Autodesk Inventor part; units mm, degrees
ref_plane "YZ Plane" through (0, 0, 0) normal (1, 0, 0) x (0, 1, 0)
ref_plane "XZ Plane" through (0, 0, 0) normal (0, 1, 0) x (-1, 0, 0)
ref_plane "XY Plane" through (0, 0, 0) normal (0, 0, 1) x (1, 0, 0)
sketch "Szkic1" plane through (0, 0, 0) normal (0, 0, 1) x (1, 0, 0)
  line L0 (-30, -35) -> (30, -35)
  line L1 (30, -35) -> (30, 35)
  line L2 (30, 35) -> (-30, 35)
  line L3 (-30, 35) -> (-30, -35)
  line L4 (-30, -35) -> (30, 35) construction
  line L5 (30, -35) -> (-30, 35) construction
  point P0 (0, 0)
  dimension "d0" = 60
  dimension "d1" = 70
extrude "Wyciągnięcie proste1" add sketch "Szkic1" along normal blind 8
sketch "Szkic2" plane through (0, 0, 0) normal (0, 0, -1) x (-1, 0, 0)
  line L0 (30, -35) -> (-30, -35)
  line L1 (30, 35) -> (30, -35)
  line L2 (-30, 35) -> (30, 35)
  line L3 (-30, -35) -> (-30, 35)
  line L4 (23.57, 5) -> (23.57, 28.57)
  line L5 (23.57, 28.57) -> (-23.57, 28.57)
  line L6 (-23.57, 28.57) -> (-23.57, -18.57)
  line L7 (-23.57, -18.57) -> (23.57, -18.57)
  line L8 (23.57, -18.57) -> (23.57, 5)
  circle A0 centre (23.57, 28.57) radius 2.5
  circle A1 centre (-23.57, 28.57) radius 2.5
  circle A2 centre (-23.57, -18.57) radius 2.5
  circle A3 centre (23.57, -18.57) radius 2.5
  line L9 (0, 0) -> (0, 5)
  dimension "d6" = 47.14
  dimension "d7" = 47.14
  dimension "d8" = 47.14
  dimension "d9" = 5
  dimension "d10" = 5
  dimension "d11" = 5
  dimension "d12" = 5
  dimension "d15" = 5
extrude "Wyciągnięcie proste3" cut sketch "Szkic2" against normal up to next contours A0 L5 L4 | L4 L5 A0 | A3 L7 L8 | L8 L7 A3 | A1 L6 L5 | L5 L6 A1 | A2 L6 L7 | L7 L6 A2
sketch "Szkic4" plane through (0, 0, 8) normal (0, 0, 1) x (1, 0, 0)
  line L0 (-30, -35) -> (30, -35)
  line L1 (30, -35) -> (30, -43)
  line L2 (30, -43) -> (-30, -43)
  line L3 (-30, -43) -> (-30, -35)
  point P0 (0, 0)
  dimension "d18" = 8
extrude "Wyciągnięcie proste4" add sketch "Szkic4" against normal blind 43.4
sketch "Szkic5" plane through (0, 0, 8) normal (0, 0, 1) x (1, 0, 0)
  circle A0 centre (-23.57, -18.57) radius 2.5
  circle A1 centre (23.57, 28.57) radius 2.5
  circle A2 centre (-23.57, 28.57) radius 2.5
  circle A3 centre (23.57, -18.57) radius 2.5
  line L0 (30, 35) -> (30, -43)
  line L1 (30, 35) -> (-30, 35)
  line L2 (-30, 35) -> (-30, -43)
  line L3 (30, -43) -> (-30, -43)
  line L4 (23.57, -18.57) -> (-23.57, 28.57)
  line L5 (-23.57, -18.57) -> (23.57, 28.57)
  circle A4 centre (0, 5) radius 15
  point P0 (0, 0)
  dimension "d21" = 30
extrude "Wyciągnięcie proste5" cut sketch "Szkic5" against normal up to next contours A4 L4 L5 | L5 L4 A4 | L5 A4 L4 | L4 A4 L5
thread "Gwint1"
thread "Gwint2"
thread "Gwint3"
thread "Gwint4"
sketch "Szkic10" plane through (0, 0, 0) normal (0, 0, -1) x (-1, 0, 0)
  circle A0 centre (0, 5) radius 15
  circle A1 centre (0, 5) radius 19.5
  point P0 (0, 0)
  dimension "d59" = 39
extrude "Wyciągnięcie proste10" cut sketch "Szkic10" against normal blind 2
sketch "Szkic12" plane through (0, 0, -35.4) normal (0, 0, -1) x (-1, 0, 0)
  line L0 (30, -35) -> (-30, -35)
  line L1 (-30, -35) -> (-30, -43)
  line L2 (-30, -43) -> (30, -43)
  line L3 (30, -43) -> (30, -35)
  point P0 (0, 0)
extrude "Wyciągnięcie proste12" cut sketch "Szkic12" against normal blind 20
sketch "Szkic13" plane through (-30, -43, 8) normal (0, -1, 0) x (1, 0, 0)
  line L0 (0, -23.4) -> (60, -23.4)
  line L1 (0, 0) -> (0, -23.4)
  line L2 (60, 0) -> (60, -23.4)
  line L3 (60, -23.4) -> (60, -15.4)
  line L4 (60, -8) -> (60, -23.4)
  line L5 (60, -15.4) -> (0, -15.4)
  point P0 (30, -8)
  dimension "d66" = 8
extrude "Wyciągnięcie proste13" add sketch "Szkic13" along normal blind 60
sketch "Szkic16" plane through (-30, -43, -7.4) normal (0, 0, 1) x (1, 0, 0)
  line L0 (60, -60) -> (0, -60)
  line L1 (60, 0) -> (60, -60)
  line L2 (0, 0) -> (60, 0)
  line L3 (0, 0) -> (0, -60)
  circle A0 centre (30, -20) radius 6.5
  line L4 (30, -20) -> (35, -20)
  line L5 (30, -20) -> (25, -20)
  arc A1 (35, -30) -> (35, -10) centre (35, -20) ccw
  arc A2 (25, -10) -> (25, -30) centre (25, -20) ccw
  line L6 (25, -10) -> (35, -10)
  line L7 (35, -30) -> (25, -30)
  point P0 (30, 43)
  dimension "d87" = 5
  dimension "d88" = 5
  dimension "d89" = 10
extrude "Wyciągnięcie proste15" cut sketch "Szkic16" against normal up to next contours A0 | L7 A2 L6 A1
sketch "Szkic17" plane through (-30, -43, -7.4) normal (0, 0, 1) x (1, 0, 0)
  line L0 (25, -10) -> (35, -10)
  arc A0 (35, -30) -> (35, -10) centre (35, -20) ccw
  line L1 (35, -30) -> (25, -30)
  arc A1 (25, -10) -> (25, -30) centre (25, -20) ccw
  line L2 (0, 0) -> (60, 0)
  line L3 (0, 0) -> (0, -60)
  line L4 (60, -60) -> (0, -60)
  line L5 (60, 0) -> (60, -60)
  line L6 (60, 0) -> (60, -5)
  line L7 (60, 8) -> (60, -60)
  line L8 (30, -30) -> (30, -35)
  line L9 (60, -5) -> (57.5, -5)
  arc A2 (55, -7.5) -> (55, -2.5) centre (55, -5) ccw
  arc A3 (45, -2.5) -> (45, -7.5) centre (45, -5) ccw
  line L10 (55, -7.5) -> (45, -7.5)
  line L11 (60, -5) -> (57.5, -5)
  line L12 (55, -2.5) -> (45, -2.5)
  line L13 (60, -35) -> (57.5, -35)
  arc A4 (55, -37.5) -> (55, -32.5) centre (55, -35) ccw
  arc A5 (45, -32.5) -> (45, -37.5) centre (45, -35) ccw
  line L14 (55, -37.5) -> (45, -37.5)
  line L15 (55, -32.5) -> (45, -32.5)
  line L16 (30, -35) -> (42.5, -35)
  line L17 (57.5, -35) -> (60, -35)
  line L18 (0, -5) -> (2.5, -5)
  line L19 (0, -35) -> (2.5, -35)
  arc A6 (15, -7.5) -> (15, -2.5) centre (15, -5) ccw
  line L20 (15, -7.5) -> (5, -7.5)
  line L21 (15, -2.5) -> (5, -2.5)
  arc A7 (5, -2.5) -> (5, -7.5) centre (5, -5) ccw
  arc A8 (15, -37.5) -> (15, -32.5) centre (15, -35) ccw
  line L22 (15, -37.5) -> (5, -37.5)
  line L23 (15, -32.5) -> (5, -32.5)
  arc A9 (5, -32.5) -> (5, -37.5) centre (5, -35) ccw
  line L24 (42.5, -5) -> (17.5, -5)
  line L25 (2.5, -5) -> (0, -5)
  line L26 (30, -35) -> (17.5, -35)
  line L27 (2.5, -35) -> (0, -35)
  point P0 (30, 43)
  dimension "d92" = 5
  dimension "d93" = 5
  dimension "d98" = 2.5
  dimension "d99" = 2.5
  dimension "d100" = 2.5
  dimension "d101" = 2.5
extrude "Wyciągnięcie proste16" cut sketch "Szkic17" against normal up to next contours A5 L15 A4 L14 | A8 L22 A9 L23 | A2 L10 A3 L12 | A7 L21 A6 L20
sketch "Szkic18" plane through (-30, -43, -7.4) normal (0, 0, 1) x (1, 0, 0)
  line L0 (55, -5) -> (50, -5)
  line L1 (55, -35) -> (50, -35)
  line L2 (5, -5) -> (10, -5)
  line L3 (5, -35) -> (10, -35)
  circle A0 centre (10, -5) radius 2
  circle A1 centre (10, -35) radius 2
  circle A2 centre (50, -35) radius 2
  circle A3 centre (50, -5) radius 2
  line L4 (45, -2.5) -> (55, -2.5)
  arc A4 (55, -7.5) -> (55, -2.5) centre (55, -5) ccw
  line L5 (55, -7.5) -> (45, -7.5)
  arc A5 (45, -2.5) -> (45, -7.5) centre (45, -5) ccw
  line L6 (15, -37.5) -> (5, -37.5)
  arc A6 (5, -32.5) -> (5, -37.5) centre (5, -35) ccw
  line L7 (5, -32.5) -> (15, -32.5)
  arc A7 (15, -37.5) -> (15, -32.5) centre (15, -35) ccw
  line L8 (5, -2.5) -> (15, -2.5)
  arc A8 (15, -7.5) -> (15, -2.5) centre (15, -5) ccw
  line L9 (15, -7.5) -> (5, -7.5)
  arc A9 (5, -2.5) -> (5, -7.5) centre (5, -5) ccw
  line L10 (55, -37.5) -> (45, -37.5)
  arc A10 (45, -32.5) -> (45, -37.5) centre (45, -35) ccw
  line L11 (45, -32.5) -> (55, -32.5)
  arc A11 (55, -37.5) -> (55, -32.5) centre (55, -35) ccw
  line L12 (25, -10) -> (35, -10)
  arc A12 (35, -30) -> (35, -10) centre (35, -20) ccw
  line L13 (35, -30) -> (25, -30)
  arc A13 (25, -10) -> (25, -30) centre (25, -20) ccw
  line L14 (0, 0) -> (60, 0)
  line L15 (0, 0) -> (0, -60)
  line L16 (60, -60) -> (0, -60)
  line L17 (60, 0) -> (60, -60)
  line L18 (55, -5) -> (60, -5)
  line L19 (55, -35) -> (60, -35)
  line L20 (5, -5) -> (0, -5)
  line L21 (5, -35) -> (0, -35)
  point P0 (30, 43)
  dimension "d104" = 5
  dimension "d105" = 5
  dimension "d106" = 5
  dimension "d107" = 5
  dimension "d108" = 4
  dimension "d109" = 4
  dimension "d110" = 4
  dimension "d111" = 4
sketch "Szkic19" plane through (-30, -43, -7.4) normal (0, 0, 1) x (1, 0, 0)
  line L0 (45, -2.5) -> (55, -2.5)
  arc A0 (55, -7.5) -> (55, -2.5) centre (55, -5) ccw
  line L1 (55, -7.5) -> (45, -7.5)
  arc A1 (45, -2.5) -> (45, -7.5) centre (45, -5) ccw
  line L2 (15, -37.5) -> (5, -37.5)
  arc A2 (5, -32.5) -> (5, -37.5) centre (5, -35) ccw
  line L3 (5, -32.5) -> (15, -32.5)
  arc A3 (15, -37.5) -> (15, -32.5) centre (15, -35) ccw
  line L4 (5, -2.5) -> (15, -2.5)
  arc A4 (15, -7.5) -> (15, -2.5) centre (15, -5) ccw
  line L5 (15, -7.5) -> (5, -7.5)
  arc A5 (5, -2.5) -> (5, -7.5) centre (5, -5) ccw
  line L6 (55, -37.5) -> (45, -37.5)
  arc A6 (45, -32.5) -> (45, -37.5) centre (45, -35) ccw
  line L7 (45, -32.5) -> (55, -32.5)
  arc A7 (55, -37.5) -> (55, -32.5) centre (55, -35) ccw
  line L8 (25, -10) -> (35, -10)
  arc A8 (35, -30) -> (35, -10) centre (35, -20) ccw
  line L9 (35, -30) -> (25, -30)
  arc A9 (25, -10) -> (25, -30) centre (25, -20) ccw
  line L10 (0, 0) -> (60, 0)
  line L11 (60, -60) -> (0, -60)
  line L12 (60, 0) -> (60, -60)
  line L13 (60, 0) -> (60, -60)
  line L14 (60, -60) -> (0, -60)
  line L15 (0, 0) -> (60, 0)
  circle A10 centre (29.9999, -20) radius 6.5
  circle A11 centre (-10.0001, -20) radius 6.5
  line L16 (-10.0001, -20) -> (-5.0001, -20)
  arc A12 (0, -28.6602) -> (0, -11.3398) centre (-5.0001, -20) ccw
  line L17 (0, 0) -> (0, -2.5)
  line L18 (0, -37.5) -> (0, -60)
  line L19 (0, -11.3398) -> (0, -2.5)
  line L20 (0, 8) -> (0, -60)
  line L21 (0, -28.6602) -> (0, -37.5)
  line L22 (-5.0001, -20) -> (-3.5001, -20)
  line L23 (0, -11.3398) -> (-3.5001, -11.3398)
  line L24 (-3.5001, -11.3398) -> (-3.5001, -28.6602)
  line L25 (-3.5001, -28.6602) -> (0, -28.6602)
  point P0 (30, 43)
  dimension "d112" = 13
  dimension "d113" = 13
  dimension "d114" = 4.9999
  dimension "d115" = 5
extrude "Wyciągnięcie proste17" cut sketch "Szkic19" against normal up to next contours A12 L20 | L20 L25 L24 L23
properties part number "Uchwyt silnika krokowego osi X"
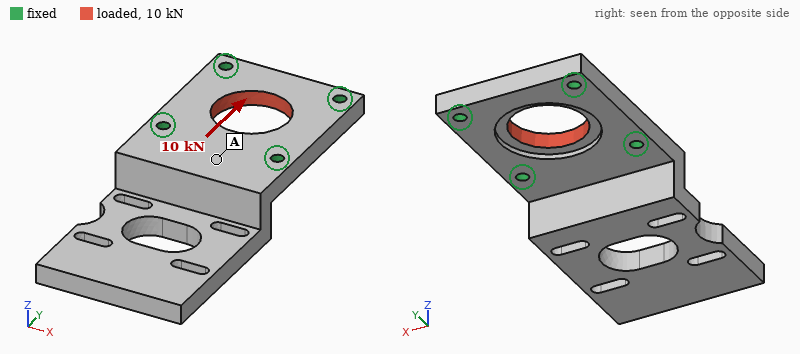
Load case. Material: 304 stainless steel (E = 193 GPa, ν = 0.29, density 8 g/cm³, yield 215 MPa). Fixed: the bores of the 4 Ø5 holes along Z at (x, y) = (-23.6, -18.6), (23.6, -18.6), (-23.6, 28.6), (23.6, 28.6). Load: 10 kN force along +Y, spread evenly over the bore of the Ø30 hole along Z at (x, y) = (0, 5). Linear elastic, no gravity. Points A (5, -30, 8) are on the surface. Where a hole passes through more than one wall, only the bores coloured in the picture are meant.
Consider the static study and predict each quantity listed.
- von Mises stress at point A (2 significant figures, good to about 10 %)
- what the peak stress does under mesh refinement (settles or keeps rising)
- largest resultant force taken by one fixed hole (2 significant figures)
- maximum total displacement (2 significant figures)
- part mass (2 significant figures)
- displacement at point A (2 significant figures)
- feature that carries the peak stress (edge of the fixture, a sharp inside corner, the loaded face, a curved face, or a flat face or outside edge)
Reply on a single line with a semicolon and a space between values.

6.8 MPa; keeps rising; 2.7 kN; 5.5 µm; 480 g; 1.5 µm; edge of the fixture
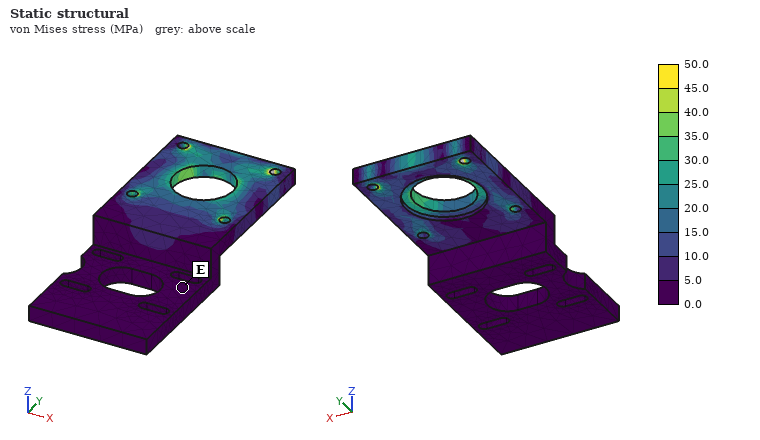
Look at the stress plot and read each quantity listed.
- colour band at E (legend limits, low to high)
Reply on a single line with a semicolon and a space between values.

0.0 to 5.0 MPa
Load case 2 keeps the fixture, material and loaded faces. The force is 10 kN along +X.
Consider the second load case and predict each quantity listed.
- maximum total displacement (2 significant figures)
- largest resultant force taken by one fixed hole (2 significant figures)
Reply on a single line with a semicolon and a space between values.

5.1 µm; 2.7 kN
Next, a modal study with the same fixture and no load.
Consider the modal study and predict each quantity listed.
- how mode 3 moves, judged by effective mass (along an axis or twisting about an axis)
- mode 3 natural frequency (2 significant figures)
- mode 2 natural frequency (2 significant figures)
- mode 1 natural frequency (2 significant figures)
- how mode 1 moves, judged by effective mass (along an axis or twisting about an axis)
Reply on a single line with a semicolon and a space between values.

along X; 2900 Hz; 2200 Hz; 670 Hz; along Z
